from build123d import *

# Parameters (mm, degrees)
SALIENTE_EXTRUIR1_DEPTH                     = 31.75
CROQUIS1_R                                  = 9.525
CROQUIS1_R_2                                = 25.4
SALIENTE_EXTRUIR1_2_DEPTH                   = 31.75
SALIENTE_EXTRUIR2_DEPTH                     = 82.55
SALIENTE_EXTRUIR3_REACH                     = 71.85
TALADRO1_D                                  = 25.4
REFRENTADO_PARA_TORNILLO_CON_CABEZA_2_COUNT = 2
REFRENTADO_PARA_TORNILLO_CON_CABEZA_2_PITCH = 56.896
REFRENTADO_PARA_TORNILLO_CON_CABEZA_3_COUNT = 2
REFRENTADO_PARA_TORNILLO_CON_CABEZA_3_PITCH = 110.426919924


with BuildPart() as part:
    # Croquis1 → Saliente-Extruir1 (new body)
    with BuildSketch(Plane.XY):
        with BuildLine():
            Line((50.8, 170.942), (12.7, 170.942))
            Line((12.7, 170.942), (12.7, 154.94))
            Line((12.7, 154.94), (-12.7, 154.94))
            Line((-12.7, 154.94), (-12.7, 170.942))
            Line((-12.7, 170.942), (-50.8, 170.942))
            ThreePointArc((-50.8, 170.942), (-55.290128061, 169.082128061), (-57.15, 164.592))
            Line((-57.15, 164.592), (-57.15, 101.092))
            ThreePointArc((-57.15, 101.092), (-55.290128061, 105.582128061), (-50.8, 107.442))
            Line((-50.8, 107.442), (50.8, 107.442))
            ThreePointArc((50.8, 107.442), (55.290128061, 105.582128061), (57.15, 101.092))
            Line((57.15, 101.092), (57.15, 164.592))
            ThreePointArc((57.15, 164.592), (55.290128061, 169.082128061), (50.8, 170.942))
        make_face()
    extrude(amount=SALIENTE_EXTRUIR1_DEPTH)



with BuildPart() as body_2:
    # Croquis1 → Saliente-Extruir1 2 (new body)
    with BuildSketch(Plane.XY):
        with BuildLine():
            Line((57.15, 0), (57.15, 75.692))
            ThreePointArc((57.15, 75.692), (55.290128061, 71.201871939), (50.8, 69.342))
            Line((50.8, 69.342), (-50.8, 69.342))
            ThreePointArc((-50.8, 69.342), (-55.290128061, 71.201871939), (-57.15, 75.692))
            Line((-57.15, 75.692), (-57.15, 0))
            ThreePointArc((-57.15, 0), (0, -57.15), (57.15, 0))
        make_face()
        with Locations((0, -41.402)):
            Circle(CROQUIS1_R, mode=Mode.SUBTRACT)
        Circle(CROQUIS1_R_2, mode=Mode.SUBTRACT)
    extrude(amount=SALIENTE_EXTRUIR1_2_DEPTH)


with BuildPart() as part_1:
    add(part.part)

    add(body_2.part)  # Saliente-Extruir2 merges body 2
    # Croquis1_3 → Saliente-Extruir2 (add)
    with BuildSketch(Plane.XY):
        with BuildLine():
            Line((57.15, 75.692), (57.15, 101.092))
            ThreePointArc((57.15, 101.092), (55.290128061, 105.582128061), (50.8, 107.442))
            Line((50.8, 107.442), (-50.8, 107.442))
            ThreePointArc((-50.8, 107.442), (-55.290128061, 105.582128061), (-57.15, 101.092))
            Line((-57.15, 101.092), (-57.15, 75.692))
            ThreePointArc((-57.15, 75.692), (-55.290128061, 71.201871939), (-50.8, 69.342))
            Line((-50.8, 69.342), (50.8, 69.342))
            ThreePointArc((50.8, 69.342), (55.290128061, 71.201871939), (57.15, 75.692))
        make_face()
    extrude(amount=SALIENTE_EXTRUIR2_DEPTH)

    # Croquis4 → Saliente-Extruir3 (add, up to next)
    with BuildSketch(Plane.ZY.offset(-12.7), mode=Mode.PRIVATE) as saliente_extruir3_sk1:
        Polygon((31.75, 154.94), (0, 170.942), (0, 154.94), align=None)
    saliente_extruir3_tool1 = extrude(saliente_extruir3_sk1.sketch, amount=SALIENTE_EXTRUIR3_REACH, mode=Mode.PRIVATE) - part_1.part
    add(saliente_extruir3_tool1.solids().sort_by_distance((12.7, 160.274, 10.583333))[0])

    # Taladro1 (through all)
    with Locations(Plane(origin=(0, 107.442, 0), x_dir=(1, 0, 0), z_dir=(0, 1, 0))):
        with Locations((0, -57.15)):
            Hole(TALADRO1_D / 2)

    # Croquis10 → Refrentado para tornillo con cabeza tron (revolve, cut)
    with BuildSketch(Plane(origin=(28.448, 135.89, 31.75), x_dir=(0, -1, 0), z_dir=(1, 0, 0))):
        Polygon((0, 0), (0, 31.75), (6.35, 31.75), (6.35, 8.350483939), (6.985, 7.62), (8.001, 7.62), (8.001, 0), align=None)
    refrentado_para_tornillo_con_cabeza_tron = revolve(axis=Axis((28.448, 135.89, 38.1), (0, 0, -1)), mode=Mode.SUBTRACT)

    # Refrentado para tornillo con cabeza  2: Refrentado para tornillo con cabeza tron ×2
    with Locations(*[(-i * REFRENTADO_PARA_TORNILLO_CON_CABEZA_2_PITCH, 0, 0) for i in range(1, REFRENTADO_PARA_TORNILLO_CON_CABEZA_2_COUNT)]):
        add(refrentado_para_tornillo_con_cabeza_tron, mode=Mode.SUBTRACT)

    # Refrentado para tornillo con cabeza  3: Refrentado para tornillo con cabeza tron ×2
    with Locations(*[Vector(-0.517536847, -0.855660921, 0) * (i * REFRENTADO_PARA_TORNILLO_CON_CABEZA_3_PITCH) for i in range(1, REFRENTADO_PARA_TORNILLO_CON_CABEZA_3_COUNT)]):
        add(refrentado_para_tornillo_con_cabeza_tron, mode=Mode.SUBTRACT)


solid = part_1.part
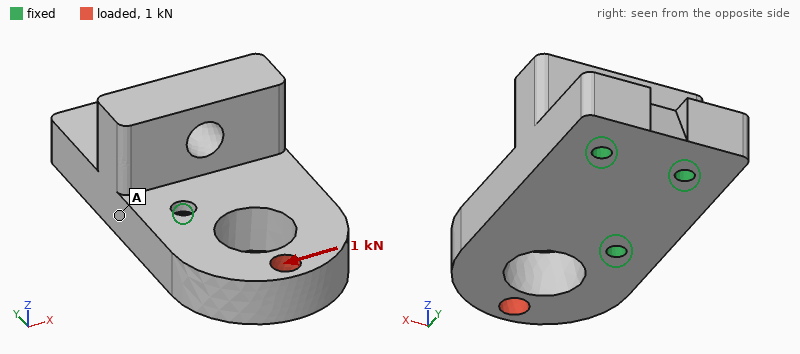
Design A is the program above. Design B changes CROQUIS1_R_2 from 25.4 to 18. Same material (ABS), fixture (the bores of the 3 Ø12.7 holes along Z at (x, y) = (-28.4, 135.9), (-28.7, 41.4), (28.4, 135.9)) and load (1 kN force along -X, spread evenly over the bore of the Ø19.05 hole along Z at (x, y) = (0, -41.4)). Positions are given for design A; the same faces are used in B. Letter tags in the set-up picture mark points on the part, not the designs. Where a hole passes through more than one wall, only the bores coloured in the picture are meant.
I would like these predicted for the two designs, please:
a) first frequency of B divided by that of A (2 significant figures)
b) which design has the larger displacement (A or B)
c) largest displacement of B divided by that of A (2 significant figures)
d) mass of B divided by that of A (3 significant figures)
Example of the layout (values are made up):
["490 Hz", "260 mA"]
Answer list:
["1.0", "A", "0.72", "1.04"]
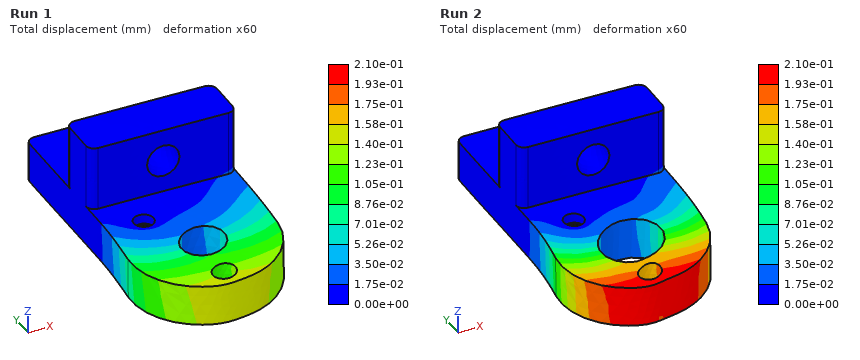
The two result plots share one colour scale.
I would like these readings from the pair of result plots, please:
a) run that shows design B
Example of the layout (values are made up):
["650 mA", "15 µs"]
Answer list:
["Run 1"]
